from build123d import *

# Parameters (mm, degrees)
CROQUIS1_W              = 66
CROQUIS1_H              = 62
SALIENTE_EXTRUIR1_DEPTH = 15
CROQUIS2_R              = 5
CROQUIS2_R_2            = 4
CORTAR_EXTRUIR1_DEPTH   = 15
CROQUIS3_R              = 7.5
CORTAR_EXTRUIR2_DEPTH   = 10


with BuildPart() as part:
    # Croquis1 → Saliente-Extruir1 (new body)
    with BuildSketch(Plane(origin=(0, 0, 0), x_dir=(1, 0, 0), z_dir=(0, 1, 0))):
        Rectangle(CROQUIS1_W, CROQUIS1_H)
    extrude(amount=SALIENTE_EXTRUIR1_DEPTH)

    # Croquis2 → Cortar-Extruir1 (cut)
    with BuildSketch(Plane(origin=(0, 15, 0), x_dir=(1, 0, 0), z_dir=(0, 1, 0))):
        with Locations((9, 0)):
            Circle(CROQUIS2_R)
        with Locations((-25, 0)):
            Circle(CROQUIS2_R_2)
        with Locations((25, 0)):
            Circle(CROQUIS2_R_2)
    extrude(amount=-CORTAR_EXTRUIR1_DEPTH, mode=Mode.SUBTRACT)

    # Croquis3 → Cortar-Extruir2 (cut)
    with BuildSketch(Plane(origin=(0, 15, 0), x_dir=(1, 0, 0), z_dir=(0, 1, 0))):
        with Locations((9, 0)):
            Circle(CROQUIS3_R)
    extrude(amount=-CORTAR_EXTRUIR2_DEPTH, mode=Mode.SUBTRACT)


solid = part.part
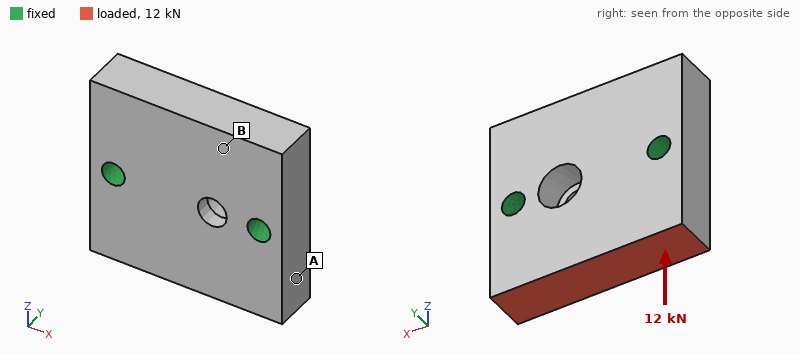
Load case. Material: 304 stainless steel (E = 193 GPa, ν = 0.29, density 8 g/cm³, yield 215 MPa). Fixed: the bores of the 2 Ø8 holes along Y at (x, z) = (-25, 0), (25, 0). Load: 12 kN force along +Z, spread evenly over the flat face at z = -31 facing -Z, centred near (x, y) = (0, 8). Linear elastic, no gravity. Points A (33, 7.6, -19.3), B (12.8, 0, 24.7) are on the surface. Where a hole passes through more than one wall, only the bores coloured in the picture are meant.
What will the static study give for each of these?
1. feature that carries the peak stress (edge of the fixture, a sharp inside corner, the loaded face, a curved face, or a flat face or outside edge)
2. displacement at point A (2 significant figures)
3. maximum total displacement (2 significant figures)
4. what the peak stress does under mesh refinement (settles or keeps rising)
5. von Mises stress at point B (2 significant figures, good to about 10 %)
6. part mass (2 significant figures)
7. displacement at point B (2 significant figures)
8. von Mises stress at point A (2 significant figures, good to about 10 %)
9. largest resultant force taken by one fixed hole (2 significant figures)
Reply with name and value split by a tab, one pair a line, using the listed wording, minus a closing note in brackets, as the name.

feature that carries the peak stress	edge of the fixture
displacement at point A	1.4 µm
maximum total displacement	3.0 µm
what the peak stress does under mesh refinement	keeps rising
von Mises stress at point B	2.8 MPa
part mass	460 g
displacement at point B	0.64 µm
von Mises stress at point A	12 MPa
largest resultant force taken by one fixed hole	6.1 kN
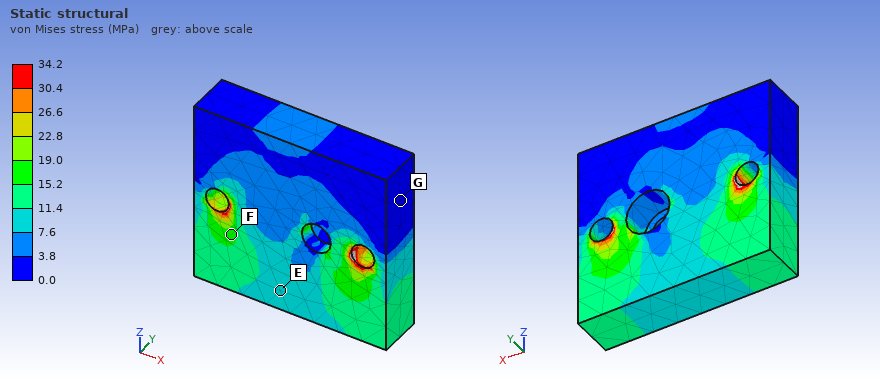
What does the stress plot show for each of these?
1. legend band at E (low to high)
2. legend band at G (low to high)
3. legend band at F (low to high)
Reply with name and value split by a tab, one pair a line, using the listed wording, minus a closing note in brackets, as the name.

legend band at E	7.6 to 11.4 MPa
legend band at G	0.0 to 3.8 MPa
legend band at F	15.2 to 19.0 MPa
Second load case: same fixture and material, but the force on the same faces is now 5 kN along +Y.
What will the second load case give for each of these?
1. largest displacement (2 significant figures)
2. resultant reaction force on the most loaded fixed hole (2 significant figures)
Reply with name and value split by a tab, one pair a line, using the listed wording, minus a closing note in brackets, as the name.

largest displacement	23 µm
resultant reaction force on the most loaded fixed hole	2.6 kN
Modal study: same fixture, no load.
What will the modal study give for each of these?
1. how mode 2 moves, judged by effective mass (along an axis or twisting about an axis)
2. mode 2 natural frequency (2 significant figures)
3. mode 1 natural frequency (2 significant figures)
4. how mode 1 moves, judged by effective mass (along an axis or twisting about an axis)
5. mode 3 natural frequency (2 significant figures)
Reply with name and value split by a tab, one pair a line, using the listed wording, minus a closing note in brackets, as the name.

how mode 2 moves, judged by effective mass	along Y
mode 2 natural frequency	10 kHz
mode 1 natural frequency	8500 Hz
how mode 1 moves, judged by effective mass	twisting about X
mode 3 natural frequency	15 kHz
